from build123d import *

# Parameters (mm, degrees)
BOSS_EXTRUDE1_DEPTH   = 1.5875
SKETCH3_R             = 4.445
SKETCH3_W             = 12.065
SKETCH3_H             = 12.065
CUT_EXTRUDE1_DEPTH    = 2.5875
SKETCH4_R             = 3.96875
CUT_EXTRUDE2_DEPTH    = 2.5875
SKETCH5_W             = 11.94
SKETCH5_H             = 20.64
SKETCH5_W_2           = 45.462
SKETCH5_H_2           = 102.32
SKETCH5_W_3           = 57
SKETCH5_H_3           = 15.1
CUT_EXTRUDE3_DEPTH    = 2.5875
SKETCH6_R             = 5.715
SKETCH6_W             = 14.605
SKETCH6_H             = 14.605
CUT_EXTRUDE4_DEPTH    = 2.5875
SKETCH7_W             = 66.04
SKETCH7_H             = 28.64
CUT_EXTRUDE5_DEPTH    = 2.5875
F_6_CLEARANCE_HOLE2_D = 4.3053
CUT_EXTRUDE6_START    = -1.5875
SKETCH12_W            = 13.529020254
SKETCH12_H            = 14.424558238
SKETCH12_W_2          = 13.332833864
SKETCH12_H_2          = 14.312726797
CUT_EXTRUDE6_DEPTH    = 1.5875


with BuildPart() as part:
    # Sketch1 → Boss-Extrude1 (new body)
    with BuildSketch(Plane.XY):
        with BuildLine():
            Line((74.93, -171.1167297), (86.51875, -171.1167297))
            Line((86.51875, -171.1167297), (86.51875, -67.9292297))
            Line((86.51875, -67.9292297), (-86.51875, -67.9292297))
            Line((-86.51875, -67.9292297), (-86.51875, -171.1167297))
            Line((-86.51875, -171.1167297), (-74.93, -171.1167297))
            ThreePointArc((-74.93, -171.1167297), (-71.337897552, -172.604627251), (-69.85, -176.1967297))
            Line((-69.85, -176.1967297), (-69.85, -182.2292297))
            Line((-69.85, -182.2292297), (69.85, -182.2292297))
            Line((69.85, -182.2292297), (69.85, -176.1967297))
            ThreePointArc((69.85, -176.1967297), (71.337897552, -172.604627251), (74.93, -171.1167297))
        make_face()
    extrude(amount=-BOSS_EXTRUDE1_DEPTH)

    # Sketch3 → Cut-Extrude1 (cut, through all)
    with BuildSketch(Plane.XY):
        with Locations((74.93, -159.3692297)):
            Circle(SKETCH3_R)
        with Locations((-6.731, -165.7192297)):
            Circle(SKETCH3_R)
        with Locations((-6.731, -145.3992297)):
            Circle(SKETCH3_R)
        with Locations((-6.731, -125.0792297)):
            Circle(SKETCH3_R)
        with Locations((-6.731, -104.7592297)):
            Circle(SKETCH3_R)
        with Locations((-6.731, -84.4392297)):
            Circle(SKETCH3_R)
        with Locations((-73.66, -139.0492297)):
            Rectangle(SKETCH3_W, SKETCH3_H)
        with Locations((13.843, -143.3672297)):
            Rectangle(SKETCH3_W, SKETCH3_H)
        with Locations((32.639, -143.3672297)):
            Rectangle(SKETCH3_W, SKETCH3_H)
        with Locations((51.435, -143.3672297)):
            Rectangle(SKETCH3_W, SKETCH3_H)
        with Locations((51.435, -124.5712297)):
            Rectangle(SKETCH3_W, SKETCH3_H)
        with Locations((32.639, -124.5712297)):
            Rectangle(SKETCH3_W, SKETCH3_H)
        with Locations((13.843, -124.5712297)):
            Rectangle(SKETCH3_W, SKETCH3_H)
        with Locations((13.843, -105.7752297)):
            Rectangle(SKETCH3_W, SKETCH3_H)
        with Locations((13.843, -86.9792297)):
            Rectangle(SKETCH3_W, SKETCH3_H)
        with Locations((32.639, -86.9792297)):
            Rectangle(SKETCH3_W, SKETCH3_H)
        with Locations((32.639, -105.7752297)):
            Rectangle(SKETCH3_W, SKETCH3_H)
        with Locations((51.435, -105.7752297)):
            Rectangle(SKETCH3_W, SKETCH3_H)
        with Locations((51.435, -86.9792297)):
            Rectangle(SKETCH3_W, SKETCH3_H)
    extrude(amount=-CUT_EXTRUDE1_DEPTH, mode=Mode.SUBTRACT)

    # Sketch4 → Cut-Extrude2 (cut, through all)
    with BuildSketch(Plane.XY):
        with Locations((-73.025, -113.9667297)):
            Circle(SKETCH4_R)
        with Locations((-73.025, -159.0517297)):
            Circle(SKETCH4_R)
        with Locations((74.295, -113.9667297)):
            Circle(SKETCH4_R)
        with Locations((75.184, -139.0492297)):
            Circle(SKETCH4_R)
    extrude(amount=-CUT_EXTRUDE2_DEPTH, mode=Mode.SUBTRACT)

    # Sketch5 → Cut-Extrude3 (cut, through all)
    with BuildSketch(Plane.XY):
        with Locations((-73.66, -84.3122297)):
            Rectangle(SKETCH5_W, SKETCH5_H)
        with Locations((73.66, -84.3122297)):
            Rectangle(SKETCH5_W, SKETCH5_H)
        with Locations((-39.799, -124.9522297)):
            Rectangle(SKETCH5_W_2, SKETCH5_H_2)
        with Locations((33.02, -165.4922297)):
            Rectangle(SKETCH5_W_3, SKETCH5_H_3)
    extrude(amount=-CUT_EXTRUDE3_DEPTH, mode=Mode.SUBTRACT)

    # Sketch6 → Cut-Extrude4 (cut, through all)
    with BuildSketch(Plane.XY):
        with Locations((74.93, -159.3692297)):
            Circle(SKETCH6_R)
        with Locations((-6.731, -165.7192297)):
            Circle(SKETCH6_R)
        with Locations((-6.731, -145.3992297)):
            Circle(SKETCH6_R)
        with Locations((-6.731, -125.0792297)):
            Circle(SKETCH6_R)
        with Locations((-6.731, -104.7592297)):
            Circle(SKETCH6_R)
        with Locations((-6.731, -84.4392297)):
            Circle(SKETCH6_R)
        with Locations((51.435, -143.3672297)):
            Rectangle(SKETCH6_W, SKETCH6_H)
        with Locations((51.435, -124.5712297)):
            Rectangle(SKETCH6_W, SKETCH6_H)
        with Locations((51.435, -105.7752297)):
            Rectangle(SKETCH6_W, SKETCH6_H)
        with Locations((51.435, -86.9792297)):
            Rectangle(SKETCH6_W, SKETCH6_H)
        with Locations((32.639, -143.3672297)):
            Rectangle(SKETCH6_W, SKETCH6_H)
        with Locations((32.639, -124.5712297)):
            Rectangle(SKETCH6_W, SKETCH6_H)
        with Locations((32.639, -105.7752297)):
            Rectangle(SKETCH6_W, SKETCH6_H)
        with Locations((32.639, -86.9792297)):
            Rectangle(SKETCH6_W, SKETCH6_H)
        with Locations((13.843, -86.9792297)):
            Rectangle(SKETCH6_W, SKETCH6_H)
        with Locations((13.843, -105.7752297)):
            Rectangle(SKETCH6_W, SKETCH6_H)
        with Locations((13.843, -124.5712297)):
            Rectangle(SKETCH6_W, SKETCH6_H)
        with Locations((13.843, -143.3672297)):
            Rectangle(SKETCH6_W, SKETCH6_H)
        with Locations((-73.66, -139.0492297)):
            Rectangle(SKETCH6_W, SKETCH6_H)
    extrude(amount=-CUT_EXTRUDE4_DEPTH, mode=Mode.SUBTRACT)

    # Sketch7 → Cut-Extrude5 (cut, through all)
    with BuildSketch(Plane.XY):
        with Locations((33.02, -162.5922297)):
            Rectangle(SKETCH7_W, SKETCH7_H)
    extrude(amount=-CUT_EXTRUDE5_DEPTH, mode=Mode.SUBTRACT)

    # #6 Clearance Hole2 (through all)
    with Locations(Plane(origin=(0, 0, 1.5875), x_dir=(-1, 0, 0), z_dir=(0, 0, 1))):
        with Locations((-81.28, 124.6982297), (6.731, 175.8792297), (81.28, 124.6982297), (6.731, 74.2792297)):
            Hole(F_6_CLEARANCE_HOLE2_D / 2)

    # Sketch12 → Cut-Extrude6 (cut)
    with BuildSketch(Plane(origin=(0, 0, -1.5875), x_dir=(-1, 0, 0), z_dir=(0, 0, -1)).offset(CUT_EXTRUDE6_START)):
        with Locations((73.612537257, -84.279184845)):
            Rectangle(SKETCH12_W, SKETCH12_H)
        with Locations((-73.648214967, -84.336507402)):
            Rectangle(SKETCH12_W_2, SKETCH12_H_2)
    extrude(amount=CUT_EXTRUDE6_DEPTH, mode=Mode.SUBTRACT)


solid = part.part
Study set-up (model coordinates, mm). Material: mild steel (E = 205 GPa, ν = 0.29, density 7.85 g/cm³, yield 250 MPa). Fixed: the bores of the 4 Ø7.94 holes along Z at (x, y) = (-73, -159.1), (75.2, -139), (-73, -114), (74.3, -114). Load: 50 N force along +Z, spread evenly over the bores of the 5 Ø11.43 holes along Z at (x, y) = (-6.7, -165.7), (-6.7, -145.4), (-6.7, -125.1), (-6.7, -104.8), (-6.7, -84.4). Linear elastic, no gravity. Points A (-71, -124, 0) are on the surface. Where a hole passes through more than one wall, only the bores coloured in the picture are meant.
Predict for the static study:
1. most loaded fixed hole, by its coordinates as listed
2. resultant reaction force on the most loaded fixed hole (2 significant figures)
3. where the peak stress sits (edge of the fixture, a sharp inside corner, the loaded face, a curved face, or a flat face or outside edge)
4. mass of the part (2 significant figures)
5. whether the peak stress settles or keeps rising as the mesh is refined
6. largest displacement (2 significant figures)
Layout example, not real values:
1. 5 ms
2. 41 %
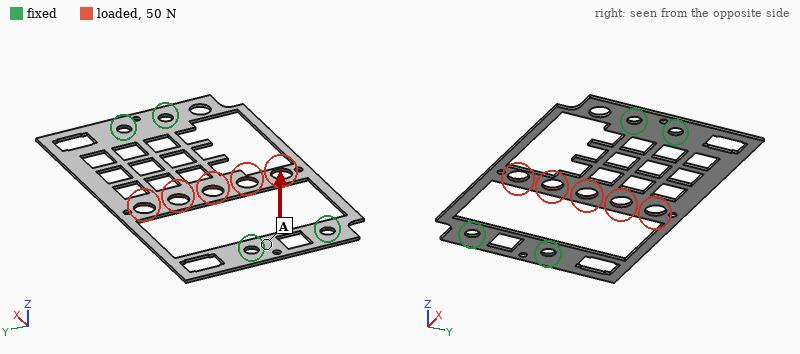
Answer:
1. (74.3, -114)
2. 19 N
3. a sharp inside corner
4. 110 g
5. keeps rising
6. 0.89 mm
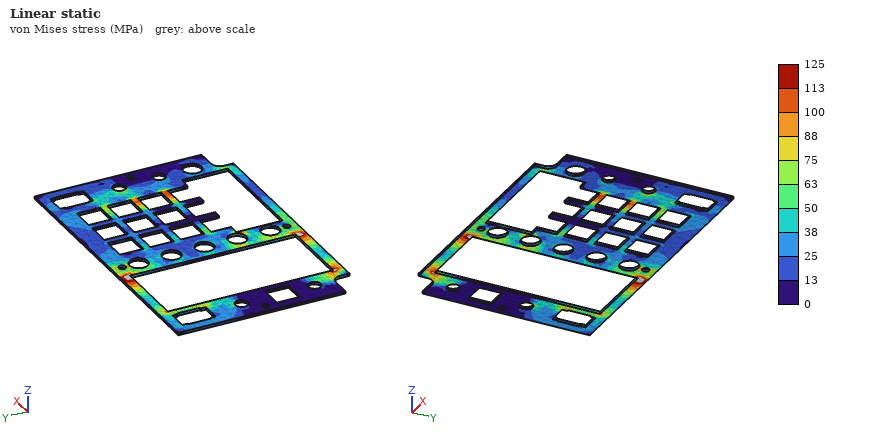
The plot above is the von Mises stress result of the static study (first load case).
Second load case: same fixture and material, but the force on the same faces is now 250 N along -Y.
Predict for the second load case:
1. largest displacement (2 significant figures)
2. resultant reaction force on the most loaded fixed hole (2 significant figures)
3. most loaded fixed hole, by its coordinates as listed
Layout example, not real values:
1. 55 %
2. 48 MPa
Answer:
1. 67 µm
2. 260 N
3. (75.2, -139)
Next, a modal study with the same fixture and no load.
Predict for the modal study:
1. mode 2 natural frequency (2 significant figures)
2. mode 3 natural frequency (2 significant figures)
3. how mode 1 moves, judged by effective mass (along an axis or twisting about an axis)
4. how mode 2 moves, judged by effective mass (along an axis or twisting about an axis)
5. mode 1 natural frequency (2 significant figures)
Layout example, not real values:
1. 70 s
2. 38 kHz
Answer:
1. 300 Hz
2. 510 Hz
3. along Z
4. twisting about X
5. 230 Hz
